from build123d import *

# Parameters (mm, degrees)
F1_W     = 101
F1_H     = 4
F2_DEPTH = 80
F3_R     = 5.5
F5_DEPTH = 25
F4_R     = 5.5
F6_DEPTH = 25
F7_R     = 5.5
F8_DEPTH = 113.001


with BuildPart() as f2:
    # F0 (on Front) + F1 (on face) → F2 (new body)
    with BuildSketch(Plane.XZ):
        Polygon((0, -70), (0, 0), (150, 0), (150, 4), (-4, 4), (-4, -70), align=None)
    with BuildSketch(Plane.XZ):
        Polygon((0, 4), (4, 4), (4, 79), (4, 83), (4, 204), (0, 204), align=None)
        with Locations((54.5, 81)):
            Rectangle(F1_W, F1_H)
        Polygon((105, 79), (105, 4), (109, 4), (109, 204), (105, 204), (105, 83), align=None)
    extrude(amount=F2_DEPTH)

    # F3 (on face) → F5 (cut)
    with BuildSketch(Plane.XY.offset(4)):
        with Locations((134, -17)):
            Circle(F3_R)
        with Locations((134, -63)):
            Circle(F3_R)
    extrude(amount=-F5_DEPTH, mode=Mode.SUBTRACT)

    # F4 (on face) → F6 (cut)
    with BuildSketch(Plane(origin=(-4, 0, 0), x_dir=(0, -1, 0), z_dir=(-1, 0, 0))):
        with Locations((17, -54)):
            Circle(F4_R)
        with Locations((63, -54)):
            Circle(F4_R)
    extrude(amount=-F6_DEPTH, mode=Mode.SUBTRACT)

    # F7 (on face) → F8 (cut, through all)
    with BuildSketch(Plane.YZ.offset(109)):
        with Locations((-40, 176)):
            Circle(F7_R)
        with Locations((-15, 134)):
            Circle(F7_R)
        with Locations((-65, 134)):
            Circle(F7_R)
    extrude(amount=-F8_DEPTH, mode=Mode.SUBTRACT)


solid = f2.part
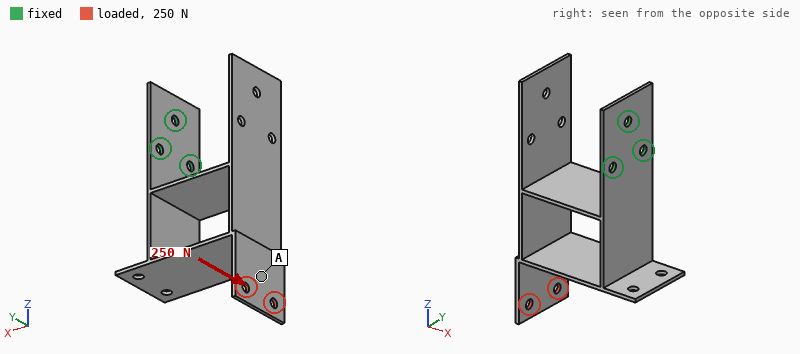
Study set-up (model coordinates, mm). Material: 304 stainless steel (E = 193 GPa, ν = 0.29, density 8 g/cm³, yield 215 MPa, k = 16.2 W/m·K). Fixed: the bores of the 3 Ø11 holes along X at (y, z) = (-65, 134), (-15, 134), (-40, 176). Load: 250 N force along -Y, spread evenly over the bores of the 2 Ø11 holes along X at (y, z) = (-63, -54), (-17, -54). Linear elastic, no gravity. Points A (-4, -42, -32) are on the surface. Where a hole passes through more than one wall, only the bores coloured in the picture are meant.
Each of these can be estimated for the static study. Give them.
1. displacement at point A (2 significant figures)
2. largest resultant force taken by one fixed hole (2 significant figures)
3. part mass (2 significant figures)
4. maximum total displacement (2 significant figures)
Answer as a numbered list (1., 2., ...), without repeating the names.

1. 1.1 mm
2. 940 N
3. 1.8 kg
4. 1.3 mm
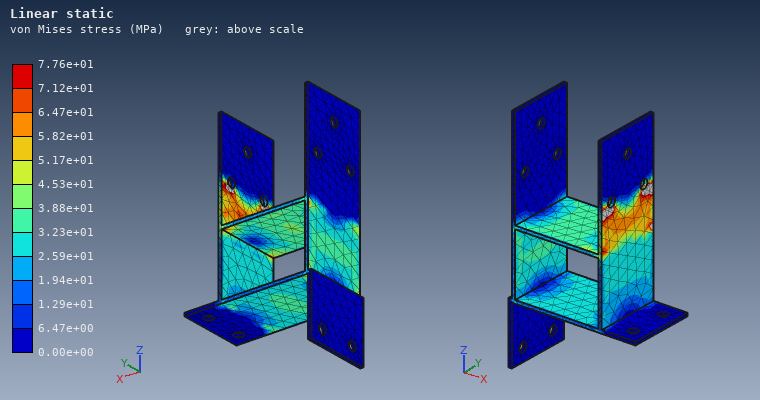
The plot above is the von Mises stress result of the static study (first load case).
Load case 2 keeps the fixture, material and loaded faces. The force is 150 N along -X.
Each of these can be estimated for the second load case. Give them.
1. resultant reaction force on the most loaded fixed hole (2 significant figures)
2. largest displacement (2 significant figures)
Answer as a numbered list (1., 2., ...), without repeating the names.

1. 110 N
2. 3.6 mm
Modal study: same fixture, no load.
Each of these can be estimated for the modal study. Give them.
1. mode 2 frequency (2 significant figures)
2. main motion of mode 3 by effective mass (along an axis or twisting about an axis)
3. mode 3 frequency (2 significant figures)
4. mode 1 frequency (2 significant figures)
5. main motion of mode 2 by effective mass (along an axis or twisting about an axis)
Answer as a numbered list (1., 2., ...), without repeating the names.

1. 120 Hz
2. along X
3. 170 Hz
4. 42 Hz
5. along Y
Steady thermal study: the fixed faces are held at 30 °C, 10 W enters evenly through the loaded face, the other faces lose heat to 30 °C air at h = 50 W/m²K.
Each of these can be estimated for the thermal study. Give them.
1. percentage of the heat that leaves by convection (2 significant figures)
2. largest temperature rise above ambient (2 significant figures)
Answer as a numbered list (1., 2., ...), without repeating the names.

1. 100 %
2. 38 K
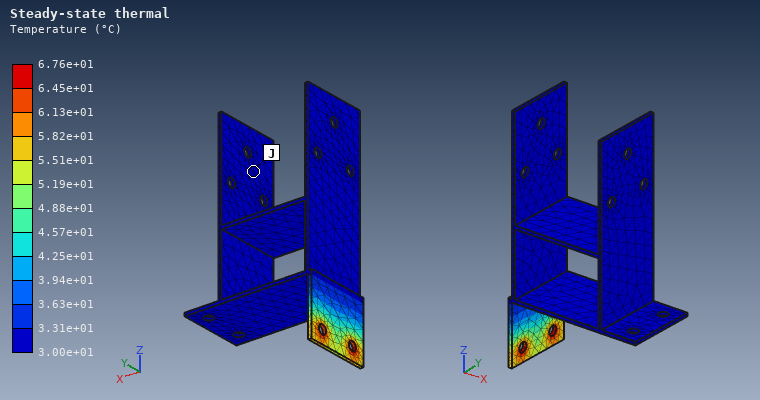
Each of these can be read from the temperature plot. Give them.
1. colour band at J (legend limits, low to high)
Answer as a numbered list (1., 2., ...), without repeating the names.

1. 3.00e+01 to 3.31e+01 °C
